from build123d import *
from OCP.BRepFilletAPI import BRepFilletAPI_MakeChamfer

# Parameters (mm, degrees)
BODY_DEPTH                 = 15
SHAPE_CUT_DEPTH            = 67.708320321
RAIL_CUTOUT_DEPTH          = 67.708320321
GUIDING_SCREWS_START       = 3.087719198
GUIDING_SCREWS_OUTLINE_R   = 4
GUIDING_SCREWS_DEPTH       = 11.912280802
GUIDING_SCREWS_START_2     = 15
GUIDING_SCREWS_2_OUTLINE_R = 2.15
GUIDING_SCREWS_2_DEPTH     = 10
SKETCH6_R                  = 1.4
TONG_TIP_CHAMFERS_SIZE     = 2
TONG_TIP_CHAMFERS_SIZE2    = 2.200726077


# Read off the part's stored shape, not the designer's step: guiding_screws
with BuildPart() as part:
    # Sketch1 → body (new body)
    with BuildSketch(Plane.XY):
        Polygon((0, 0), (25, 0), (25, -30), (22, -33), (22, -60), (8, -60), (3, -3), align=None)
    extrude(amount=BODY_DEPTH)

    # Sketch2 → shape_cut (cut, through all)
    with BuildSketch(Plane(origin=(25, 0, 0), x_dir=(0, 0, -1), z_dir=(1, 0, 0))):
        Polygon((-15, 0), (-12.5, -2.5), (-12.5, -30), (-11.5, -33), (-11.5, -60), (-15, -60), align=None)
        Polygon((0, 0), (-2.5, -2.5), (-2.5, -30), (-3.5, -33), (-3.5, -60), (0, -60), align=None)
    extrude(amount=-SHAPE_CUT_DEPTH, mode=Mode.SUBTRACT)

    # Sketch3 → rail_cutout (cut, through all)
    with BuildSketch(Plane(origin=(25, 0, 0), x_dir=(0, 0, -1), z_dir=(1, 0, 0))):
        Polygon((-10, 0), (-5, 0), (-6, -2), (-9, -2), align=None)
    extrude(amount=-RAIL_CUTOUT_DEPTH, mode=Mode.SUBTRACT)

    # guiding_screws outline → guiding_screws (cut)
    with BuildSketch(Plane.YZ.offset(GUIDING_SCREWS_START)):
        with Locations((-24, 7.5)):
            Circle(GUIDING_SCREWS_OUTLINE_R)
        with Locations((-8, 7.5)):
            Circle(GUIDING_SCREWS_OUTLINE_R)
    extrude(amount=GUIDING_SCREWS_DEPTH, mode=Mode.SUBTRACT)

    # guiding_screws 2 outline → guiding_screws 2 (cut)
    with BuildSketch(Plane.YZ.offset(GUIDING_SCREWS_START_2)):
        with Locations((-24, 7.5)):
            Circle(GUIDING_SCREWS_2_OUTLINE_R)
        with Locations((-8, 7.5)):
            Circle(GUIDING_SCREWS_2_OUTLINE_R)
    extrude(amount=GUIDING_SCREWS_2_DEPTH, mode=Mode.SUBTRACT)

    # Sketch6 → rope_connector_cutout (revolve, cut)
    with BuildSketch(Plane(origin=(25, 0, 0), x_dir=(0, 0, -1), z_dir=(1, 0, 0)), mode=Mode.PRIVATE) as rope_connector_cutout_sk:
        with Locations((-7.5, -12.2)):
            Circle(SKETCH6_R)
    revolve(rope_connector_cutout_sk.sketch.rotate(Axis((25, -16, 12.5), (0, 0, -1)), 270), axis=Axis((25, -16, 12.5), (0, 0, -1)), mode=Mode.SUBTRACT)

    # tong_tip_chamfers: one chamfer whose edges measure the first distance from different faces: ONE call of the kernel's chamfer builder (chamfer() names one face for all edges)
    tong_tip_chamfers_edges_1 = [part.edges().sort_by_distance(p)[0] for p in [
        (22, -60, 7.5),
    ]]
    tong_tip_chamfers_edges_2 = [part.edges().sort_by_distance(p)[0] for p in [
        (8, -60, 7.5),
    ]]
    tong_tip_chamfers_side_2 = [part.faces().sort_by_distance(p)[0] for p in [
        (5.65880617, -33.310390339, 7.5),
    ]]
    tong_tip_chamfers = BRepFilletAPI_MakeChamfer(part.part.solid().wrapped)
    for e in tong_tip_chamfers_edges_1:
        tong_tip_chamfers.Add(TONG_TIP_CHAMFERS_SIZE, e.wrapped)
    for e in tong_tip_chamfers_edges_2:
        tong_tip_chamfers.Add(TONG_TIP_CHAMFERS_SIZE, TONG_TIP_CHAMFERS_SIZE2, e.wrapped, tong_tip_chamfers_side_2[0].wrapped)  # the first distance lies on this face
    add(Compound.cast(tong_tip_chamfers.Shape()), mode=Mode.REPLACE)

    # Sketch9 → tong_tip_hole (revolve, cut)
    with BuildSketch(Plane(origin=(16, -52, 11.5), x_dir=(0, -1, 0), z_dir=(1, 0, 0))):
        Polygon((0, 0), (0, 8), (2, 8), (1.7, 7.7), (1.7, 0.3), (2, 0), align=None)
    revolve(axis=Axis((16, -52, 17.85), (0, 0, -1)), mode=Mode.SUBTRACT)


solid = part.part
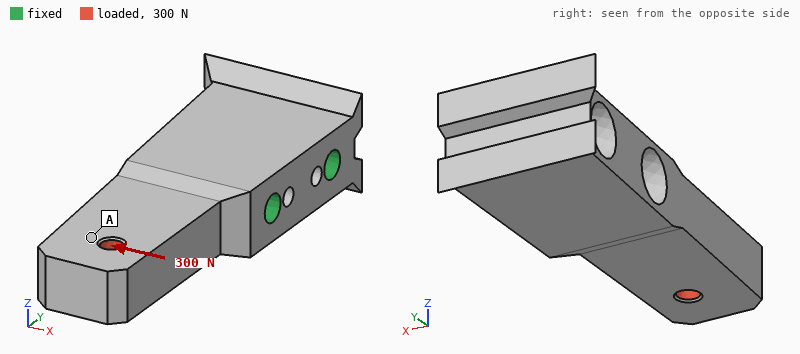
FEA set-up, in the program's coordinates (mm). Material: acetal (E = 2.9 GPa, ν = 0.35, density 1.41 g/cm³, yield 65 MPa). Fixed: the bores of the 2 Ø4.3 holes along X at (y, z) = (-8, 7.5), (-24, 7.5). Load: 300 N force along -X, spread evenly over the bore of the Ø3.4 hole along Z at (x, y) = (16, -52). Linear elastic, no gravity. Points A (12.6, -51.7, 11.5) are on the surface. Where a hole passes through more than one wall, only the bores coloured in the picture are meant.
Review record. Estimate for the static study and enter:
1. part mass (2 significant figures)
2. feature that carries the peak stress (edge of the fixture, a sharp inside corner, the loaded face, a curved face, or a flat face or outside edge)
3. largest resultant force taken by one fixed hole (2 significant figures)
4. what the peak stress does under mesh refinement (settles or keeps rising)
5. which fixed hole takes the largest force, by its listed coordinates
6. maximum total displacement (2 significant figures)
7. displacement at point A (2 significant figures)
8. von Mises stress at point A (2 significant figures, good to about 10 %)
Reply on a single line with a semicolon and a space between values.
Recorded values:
12 g; a sharp inside corner; 550 N; keeps rising; (-24, 7.5); 0.60 mm; 0.43 mm; 5.7 MPa
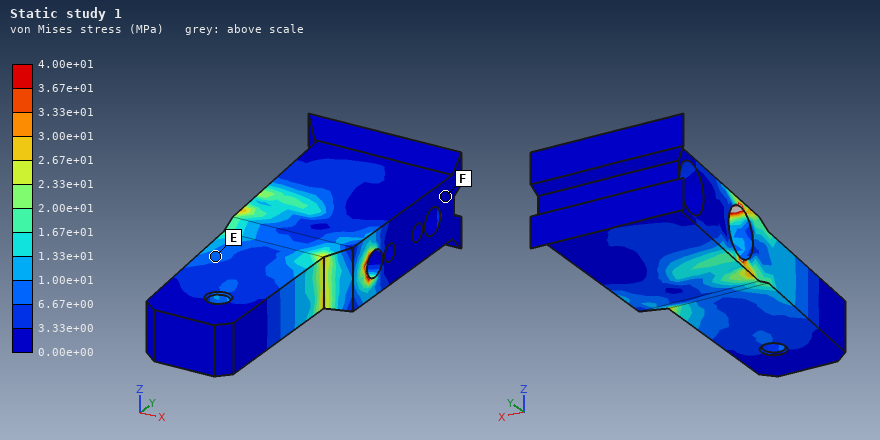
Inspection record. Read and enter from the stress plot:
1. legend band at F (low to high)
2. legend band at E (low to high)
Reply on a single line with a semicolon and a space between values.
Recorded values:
0.00e+00 to 3.33e+00 MPa; 6.67e+00 to 1.00e+01 MPa
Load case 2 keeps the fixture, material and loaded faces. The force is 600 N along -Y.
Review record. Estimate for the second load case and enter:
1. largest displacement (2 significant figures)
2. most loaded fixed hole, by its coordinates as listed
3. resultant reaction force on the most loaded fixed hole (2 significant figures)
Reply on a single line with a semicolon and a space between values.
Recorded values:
74 µm; (-24, 7.5); 510 N
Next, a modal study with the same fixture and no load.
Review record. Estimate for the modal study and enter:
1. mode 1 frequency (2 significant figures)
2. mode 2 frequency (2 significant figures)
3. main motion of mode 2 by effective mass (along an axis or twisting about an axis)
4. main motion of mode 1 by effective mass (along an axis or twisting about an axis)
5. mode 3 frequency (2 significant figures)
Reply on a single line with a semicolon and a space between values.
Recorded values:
1600 Hz; 2400 Hz; along X; along Z; 4700 Hz
